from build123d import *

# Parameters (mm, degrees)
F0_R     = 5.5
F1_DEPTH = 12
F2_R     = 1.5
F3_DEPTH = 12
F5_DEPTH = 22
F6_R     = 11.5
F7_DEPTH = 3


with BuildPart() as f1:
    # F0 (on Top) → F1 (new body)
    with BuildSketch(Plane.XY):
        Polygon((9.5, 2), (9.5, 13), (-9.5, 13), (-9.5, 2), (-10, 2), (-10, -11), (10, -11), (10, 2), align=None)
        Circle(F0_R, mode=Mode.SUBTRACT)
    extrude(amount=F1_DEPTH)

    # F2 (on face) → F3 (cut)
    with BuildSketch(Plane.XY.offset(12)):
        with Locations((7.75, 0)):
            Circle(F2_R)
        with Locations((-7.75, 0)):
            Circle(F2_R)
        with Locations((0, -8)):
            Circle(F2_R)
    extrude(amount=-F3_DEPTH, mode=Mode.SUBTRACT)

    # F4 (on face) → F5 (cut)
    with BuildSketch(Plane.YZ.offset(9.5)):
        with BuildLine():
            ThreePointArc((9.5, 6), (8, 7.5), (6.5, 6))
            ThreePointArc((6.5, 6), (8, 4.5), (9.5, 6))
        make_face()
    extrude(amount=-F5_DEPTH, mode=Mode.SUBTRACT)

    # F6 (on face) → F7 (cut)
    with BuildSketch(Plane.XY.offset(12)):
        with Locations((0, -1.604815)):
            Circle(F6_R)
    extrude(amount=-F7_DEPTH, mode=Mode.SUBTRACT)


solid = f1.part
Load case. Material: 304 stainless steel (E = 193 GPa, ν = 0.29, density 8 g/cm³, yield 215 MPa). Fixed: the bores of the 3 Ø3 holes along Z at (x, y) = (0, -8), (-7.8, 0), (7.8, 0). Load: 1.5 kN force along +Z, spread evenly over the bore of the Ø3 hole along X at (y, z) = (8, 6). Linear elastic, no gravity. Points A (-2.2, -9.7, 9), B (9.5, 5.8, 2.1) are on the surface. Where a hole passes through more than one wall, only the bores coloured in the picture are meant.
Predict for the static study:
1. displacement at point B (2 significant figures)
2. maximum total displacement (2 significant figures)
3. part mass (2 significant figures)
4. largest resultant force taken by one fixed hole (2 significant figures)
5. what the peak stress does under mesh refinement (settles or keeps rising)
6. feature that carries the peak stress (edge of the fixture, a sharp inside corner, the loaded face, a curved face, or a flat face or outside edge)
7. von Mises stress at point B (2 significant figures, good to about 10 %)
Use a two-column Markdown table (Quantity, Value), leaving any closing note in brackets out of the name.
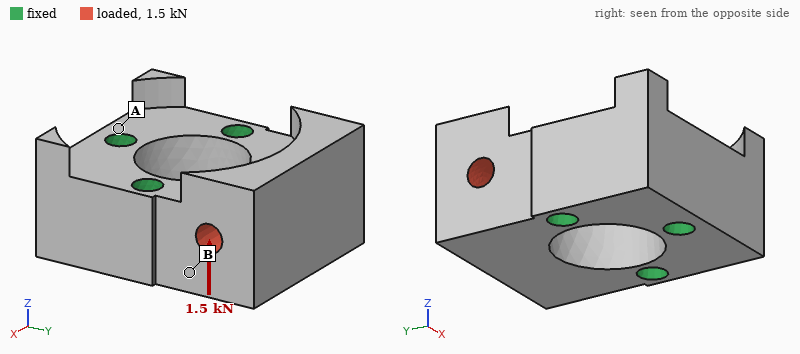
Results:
| Quantity | Value |
|---|---|
| displacement at point B | 1.9 µm |
| maximum total displacement | 6.2 µm |
| part mass | 27 g |
| largest resultant force taken by one fixed hole | 750 N |
| what the peak stress does under mesh refinement | keeps rising |
| feature that carries the peak stress | edge of the fixture |
| von Mises stress at point B | 28 MPa |
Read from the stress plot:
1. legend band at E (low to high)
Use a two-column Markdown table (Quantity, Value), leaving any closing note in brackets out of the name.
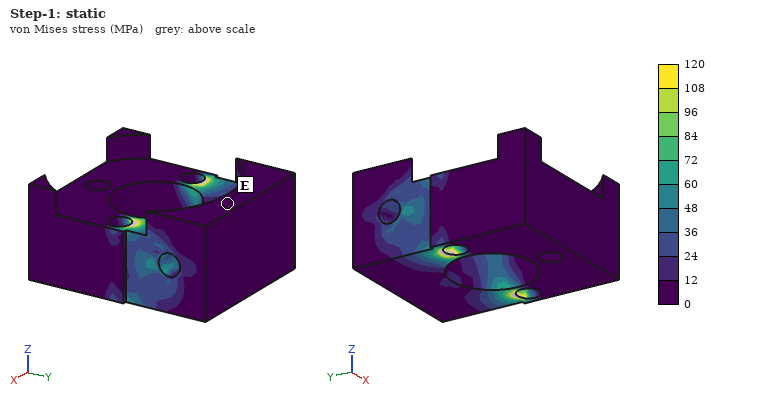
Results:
| Quantity | Value |
|---|---|
| legend band at E | 0 to 12 MPa |
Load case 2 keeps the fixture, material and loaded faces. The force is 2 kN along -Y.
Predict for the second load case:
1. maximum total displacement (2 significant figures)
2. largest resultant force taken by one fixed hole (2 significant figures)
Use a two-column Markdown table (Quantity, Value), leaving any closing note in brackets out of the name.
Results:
| Quantity | Value |
|---|---|
| maximum total displacement | 3.0 µm |
| largest resultant force taken by one fixed hole | 1.0 kN |
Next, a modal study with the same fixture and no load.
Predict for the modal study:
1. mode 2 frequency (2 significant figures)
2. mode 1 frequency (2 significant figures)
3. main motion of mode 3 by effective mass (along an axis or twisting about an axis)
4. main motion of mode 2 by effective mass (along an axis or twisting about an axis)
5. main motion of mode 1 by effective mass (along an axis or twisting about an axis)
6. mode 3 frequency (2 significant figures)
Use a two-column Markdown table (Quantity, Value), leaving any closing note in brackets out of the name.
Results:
| Quantity | Value |
|---|---|
| mode 2 frequency | 32 kHz |
| mode 1 frequency | 23 kHz |
| main motion of mode 3 by effective mass | along X |
| main motion of mode 2 by effective mass | along X |
| main motion of mode 1 by effective mass | along Z |
| mode 3 frequency | 39 kHz |
